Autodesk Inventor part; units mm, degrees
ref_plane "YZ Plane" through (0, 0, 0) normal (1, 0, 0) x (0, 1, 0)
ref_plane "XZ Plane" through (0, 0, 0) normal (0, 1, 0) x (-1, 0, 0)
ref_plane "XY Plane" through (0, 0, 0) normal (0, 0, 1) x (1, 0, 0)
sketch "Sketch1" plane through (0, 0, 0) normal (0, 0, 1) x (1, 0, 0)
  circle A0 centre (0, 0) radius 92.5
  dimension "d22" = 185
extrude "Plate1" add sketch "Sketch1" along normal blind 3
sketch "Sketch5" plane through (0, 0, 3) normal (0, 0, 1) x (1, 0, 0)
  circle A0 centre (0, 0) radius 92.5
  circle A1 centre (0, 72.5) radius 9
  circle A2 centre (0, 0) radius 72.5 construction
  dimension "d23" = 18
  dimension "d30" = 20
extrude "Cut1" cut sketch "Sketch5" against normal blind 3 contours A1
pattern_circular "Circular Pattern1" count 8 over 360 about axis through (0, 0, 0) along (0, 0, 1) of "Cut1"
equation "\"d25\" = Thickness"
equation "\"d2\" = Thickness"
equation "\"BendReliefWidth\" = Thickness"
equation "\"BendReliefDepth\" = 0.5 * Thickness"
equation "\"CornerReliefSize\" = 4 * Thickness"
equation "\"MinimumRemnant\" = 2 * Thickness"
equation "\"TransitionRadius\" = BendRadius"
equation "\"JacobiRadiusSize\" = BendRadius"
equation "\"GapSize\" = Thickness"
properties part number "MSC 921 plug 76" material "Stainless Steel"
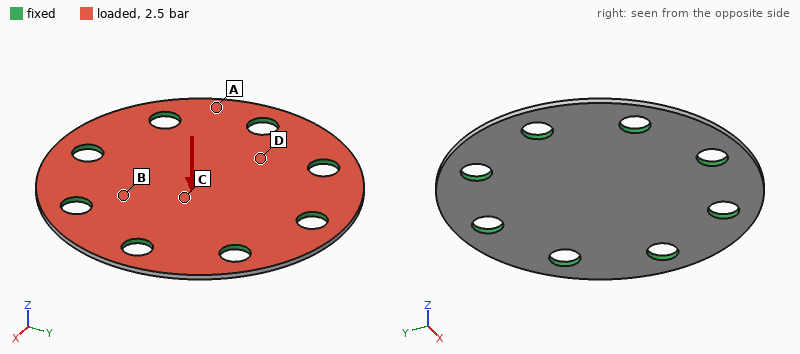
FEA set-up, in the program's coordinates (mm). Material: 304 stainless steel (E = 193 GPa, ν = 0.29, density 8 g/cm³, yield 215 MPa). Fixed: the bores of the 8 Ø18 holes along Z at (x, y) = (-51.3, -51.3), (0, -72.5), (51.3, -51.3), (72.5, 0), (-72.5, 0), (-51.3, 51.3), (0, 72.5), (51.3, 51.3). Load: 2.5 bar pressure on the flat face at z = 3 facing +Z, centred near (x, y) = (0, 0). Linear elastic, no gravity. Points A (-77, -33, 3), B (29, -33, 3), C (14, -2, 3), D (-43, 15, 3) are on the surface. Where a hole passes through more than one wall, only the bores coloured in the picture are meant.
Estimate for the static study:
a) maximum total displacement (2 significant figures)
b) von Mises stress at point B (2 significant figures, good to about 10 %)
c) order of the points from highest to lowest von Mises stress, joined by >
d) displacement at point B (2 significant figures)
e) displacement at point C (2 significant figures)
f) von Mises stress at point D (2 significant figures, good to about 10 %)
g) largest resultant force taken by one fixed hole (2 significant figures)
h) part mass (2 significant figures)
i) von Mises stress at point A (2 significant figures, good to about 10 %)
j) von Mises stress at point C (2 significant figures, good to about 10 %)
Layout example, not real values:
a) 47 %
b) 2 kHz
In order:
a) 0.17 mm
b) 18 MPa
c) C > D > B > A
d) 0.055 mm
e) 0.15 mm
f) 37 MPa
g) 780 N
h) 600 g
i) 10 MPa
j) 54 MPa
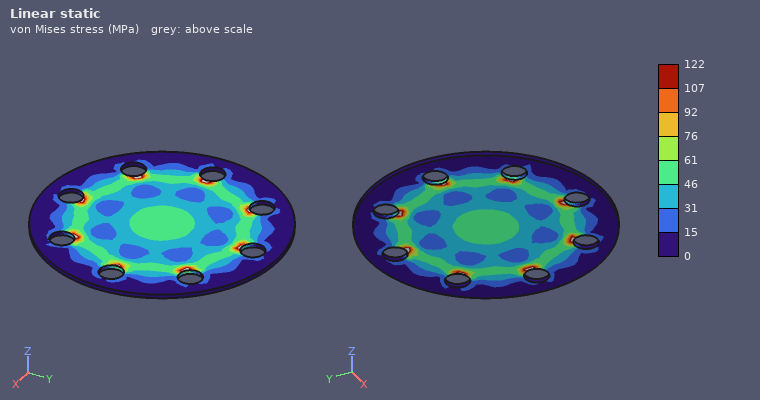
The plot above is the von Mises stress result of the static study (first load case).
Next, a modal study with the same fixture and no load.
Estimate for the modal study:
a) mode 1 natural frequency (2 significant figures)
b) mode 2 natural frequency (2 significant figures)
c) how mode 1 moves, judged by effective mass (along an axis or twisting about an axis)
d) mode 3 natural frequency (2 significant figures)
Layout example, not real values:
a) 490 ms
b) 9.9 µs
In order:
a) 1600 Hz
b) 3300 Hz
c) along Z
d) 3300 Hz
